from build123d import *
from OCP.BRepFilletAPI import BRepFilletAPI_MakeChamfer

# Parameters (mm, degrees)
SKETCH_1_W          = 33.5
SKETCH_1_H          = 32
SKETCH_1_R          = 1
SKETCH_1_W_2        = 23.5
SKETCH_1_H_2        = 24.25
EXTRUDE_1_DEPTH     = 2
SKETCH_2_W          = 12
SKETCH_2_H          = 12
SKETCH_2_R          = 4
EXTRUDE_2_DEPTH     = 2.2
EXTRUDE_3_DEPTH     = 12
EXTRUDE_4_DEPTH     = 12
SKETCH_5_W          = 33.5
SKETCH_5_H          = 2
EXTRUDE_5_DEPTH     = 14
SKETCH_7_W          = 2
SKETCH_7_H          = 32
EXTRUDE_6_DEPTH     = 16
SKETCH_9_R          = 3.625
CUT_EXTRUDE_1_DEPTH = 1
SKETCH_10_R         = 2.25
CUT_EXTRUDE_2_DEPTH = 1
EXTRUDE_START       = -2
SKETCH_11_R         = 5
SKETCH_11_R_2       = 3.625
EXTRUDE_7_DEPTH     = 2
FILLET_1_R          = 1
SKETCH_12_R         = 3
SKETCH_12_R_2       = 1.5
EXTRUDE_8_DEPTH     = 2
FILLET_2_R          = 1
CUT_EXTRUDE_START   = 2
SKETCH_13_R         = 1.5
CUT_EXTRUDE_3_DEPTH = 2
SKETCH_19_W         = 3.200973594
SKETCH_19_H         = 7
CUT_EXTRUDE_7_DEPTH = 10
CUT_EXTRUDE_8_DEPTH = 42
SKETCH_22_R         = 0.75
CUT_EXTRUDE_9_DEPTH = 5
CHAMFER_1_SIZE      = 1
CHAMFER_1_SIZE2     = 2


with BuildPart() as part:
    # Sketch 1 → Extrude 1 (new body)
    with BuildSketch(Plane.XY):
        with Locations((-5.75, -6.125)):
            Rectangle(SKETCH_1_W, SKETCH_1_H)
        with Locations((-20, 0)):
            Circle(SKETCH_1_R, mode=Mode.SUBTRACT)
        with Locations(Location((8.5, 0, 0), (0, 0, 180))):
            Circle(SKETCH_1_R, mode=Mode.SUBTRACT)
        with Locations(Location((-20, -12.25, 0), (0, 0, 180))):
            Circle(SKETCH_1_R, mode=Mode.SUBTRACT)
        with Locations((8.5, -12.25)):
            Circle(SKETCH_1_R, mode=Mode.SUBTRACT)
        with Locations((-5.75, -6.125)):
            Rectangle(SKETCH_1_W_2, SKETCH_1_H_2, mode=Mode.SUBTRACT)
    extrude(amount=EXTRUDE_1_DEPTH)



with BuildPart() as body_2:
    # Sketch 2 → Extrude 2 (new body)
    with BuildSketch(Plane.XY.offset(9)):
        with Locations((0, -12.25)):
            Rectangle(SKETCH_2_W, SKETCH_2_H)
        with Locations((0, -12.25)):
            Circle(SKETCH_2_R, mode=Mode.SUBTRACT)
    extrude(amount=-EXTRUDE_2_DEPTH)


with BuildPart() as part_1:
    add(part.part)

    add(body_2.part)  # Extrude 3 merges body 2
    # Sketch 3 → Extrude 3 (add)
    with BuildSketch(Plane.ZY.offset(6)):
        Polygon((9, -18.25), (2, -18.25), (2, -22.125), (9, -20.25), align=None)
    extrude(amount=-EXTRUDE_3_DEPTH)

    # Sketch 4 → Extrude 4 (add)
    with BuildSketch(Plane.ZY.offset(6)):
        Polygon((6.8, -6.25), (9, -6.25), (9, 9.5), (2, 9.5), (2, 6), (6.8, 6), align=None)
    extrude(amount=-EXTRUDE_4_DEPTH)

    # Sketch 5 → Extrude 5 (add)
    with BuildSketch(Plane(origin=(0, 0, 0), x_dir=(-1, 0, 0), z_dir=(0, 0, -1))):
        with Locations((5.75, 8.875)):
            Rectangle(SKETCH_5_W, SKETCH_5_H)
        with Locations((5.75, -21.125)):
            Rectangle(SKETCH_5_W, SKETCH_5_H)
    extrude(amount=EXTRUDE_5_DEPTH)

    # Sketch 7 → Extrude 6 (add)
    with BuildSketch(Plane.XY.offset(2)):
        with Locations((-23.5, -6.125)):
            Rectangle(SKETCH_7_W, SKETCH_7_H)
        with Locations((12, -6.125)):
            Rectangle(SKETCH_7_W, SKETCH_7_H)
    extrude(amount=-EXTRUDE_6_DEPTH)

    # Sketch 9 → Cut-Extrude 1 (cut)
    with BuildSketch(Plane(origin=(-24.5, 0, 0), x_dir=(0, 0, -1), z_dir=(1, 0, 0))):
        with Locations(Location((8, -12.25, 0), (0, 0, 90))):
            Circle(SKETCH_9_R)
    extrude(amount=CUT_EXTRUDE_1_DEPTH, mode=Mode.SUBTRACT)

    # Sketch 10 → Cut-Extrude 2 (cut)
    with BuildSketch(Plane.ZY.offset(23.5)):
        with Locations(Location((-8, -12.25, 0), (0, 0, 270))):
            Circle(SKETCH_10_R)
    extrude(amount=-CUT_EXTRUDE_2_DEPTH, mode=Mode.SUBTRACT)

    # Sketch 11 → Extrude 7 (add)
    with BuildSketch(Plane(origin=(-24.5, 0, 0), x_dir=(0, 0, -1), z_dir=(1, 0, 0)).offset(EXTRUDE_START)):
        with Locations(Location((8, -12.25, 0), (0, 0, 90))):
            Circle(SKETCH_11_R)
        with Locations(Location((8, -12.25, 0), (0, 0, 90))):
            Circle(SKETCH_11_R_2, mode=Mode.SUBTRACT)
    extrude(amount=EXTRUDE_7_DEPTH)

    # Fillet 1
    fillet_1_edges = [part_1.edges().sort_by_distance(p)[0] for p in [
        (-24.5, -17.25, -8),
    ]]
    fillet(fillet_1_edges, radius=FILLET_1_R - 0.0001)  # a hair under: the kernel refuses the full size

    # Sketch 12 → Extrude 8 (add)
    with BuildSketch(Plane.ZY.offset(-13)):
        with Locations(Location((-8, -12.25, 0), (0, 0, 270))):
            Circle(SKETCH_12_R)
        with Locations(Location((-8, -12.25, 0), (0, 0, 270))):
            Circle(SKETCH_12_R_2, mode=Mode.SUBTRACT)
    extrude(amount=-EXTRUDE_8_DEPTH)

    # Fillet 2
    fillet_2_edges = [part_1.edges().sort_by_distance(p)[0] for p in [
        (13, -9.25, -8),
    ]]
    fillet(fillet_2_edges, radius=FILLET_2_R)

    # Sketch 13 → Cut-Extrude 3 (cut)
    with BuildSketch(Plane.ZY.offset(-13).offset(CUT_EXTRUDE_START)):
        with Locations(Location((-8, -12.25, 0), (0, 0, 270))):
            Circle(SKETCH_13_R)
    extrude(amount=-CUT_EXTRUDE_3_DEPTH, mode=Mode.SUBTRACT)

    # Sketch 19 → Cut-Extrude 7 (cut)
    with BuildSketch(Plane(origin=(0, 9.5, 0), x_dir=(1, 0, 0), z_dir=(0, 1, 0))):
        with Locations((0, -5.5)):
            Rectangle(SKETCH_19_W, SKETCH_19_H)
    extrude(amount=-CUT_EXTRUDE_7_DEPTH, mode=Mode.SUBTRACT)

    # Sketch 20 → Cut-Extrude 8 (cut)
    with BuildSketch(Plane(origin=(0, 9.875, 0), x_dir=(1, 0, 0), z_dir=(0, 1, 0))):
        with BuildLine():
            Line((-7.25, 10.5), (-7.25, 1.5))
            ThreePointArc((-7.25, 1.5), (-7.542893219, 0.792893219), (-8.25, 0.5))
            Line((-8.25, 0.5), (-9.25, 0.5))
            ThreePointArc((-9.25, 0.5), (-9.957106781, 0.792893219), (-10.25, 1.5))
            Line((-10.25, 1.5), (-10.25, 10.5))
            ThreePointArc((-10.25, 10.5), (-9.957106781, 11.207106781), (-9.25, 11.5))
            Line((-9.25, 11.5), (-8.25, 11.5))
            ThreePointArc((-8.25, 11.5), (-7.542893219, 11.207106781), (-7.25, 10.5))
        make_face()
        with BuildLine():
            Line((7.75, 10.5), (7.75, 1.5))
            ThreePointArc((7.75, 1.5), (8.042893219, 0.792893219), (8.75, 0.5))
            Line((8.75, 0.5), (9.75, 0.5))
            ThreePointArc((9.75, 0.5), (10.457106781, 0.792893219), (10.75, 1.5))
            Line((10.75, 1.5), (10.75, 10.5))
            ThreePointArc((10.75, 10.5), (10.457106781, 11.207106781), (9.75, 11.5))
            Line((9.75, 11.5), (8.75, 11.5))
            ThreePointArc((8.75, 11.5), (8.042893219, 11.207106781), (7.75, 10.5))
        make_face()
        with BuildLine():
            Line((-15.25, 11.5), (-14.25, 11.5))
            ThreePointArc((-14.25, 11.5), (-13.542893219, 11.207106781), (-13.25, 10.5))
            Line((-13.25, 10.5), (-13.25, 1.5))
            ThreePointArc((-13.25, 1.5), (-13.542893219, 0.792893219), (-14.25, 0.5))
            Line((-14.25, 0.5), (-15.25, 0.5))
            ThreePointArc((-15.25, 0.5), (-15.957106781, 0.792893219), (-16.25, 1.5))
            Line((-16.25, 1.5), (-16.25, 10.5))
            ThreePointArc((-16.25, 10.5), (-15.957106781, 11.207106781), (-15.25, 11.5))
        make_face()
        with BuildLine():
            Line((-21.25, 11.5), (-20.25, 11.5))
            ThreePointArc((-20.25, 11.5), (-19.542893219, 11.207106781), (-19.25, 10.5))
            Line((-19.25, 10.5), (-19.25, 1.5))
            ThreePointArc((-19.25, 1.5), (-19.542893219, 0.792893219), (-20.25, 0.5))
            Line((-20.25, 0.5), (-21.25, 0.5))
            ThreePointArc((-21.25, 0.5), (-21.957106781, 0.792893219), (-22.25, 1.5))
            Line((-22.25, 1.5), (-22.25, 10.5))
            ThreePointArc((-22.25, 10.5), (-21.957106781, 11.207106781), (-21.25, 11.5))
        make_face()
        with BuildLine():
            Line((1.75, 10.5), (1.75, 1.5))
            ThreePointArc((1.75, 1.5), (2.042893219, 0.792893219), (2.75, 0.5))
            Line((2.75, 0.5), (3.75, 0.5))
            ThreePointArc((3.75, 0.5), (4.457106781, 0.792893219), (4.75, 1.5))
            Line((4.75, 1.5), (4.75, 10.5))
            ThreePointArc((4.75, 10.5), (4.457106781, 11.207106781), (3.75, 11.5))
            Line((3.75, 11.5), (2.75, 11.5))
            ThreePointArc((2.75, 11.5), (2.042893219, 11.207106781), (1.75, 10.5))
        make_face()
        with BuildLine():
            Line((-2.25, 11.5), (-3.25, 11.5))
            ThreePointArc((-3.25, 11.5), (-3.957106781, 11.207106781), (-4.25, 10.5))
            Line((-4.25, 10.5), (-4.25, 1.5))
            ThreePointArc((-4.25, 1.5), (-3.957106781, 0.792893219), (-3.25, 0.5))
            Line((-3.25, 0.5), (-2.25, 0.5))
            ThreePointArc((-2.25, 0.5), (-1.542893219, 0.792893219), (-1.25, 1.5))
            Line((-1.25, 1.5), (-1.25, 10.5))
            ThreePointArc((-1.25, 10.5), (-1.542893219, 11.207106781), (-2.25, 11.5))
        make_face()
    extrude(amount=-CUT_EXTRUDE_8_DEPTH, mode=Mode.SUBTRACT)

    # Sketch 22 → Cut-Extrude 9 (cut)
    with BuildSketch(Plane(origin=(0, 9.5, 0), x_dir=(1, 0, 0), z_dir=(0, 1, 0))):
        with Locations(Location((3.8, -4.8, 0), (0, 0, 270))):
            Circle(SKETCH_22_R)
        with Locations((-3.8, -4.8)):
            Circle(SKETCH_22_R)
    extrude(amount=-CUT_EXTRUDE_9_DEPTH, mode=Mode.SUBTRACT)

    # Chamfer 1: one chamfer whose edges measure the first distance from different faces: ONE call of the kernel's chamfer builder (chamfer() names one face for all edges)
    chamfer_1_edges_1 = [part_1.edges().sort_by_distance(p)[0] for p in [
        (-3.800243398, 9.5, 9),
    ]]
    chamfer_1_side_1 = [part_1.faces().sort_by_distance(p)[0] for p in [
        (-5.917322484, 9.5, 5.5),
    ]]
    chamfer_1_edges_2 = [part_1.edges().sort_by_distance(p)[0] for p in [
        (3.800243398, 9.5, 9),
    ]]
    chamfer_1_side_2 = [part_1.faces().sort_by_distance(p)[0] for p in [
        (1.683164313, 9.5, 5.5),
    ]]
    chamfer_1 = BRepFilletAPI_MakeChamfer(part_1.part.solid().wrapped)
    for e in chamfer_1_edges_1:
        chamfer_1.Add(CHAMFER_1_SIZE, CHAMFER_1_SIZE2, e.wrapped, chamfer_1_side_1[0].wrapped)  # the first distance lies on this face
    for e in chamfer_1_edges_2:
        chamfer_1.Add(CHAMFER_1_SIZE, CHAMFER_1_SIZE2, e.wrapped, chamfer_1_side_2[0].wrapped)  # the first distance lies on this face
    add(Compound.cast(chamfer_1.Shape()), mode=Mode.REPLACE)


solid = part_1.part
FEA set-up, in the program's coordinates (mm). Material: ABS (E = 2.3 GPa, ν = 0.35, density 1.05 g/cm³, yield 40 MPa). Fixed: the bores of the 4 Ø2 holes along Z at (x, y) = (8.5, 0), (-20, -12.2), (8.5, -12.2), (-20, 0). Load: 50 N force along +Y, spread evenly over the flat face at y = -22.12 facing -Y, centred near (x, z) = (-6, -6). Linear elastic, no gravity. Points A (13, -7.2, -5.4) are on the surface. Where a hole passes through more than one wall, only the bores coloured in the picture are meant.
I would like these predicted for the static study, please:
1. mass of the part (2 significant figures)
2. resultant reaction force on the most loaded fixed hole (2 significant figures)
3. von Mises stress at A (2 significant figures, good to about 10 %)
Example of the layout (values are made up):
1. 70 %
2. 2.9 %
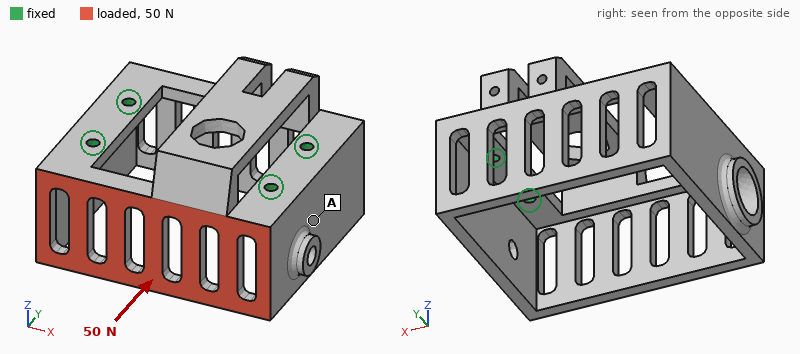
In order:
1. 5.4 g
2. 28 N
3. 1.3 MPa
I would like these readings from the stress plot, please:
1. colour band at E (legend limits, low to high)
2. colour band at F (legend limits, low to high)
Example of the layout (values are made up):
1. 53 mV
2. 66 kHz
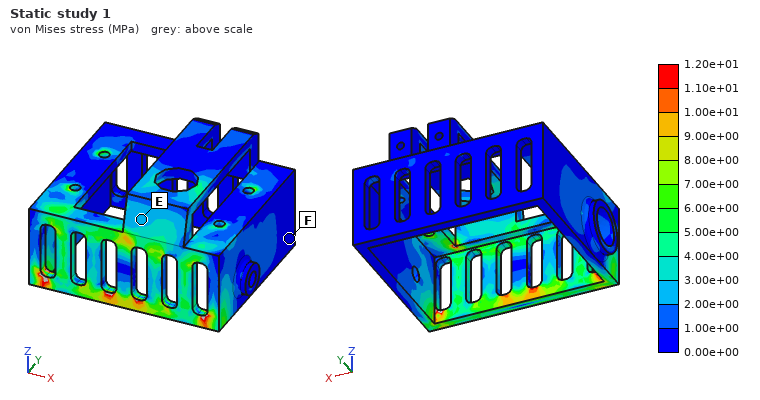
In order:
1. 2.00e+00 to 3.00e+00 MPa
2. 0.00e+00 to 1.00e+00 MPa
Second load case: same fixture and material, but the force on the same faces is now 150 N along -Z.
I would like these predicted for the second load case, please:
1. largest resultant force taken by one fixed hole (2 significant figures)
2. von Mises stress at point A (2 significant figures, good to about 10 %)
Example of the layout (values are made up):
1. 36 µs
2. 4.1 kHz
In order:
1. 120 N
2. 4.6 MPa
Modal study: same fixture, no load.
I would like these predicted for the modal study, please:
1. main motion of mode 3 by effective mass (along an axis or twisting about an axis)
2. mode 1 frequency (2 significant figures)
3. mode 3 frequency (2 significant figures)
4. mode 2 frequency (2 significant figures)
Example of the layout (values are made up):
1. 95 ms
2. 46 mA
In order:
1. along X
2. 2000 Hz
3. 2500 Hz
4. 2300 Hz
